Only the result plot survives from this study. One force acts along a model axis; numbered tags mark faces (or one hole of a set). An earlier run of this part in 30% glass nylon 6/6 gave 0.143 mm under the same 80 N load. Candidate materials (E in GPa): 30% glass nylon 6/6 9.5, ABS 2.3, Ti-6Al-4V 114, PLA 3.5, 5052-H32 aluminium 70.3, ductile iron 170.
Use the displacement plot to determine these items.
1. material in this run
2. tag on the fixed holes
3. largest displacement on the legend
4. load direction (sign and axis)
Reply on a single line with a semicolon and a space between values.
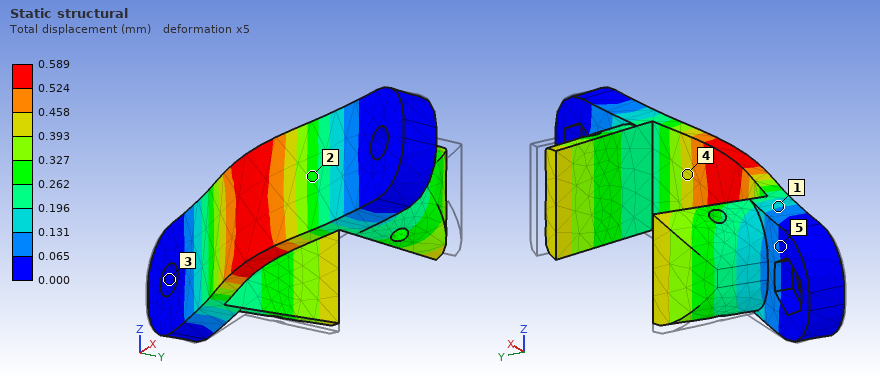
ABS; 3; 0.589 mm; -Y
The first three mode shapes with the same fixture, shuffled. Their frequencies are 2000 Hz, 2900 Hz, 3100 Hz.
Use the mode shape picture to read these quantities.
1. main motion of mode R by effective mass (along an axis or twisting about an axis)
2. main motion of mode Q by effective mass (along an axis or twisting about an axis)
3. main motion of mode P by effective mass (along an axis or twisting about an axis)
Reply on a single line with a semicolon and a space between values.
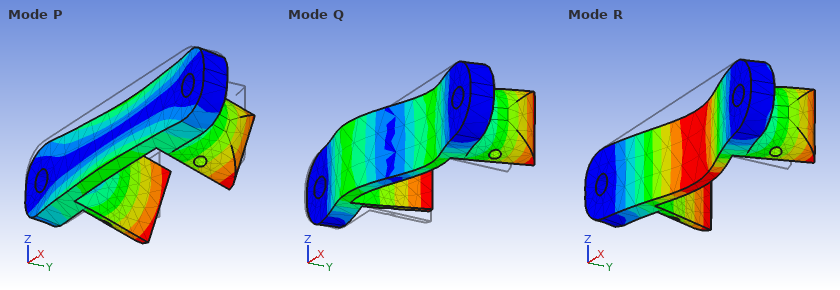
along Y; along X; along Z
